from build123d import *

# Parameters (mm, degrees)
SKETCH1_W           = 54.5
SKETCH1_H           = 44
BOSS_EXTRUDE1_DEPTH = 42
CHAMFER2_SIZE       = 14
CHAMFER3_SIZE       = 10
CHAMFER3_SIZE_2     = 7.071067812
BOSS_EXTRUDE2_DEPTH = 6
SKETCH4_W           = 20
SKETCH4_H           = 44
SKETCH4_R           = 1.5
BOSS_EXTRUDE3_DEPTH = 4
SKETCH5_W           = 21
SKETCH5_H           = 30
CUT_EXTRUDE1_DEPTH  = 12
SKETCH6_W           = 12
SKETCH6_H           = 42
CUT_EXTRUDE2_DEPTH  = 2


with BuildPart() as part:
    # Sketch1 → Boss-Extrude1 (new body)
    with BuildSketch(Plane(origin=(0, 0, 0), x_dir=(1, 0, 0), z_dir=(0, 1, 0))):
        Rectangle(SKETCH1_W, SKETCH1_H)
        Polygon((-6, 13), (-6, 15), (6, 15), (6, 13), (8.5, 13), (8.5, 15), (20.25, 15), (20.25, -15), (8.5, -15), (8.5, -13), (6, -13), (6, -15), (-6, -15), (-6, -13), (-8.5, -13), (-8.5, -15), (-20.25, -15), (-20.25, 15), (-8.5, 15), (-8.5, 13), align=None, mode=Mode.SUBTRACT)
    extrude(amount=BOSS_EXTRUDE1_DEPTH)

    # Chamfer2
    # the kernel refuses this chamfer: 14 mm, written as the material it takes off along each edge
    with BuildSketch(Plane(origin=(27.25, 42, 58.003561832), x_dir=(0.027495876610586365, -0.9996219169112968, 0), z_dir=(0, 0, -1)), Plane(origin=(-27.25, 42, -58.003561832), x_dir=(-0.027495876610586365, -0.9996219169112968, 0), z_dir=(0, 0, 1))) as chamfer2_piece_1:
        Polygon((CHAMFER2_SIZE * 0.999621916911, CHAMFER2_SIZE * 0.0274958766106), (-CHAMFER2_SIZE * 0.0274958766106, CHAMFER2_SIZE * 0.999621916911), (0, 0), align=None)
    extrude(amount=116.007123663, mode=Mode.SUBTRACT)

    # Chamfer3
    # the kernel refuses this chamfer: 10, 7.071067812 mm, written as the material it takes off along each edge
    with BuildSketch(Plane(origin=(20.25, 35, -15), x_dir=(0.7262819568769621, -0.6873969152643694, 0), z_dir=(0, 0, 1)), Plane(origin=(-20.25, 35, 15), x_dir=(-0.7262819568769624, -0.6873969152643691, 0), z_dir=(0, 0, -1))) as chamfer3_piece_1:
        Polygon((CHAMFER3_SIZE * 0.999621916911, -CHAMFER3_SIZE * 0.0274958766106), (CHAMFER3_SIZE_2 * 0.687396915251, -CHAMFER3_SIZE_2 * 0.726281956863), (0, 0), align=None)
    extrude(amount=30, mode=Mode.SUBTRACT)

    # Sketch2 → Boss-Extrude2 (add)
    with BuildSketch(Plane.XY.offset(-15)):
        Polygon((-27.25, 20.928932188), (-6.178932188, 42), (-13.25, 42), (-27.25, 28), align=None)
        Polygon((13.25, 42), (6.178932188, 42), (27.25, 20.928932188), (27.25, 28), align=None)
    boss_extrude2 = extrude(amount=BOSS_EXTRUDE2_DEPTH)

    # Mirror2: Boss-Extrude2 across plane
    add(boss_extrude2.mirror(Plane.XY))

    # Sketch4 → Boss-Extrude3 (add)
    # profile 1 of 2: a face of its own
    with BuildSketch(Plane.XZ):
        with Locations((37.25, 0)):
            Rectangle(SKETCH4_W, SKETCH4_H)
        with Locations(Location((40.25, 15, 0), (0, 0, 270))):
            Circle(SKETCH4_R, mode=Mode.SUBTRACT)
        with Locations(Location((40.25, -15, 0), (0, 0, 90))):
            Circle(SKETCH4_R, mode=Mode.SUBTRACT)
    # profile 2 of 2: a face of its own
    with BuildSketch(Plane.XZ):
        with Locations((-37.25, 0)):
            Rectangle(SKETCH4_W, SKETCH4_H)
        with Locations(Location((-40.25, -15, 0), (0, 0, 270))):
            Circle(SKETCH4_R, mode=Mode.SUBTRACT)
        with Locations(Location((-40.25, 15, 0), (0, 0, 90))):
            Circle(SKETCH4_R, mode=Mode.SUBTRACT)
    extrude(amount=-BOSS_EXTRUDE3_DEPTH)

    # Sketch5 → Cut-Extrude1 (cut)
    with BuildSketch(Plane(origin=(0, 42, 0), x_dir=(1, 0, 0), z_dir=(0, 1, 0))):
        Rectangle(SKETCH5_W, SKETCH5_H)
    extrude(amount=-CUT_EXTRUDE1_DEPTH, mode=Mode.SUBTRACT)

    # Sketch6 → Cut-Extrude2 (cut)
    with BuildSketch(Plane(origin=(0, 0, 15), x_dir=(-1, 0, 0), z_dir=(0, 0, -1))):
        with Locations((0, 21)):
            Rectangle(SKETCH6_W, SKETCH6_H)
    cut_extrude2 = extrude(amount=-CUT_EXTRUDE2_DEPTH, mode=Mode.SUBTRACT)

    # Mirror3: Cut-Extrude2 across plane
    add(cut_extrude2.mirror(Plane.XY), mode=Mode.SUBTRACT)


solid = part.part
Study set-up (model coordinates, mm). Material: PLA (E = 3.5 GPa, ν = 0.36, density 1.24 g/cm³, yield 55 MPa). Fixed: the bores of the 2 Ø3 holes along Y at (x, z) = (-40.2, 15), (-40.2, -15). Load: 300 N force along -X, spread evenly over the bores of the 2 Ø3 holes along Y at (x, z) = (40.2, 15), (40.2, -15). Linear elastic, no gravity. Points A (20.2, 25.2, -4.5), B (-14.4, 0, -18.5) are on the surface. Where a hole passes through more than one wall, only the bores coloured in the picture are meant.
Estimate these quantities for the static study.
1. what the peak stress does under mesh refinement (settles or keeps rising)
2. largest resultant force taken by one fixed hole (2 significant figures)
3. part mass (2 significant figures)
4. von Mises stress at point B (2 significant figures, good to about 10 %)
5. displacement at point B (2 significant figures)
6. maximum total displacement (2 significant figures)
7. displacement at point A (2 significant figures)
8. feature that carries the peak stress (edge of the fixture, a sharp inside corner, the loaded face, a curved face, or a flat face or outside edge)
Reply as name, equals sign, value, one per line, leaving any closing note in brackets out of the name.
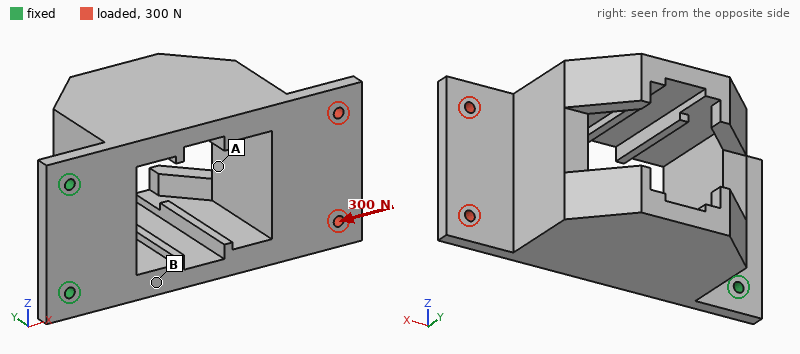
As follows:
what the peak stress does under mesh refinement = keeps rising
largest resultant force taken by one fixed hole = 150 N
part mass = 60 g
von Mises stress at point B = 2.8 MPa
displacement at point B = 0.034 mm
maximum total displacement = 0.20 mm
displacement at point A = 0.083 mm
feature that carries the peak stress = edge of the fixture
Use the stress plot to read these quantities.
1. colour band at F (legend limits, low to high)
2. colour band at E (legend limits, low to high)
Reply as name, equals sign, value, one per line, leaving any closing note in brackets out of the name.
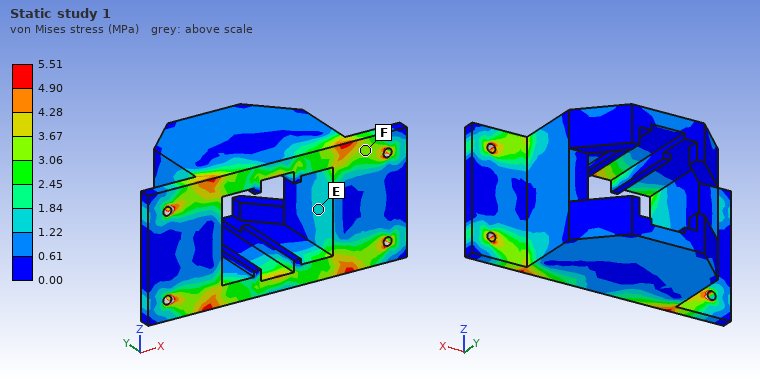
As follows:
colour band at F = 3.06 to 3.67 MPa
colour band at E = 1.22 to 1.84 MPa
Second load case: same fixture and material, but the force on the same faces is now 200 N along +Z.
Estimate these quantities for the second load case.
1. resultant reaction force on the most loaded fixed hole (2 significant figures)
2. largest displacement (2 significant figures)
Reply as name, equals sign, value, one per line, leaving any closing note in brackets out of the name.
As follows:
resultant reaction force on the most loaded fixed hole = 530 N
largest displacement = 1.2 mm
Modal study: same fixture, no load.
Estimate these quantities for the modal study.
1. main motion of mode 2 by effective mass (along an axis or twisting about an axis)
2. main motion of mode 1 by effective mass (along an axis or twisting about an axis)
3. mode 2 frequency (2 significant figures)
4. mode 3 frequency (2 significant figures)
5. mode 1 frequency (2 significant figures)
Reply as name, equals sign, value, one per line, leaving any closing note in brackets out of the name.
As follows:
main motion of mode 2 by effective mass = along Z
main motion of mode 1 by effective mass = along Y
mode 2 frequency = 480 Hz
mode 3 frequency = 560 Hz
mode 1 frequency = 100 Hz
